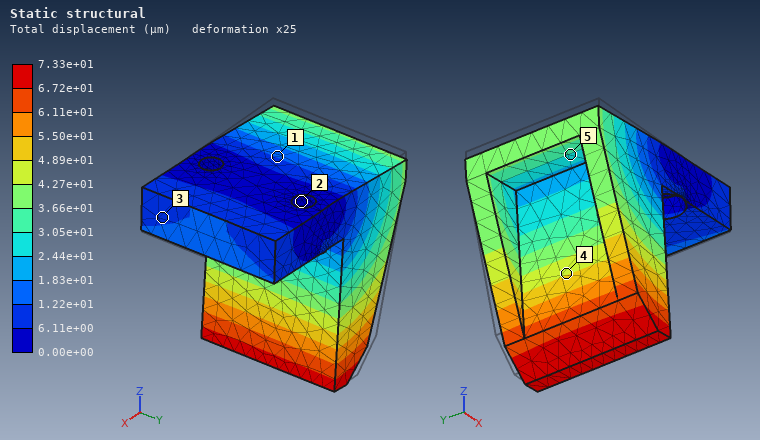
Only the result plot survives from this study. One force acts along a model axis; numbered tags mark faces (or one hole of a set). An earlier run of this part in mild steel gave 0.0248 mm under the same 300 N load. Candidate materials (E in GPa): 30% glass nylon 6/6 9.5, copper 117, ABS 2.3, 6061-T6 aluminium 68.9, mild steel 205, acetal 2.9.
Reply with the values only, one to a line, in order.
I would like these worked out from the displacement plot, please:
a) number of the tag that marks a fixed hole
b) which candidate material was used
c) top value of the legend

2
6061-T6 aluminium
7.33e+01 µm
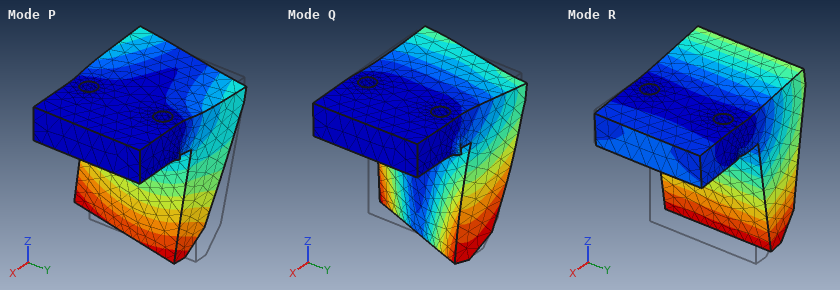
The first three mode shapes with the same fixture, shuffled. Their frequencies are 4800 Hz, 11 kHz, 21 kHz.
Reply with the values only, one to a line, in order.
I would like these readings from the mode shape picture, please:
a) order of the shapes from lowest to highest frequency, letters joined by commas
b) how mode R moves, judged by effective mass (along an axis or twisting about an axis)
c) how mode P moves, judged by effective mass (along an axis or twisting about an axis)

R, P, Q
along X
along Y
